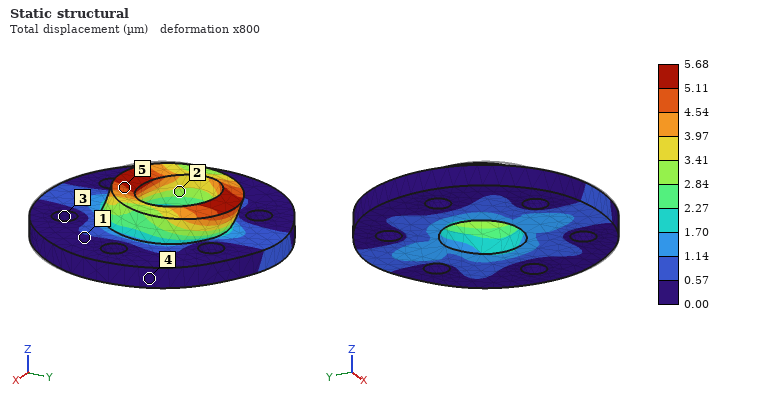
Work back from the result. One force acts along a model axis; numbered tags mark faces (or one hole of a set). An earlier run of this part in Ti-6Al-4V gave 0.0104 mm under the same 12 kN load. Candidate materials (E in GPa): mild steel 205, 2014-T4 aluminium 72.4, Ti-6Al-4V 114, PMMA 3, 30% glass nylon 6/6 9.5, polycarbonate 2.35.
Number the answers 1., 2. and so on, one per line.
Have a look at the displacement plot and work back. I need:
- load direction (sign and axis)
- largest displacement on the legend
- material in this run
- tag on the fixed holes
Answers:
1. +Y
2. 5.68 µm
3. mild steel
4. 3
